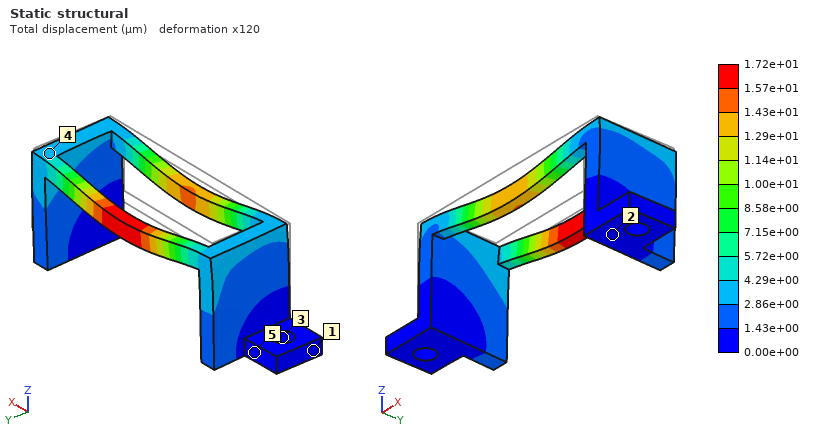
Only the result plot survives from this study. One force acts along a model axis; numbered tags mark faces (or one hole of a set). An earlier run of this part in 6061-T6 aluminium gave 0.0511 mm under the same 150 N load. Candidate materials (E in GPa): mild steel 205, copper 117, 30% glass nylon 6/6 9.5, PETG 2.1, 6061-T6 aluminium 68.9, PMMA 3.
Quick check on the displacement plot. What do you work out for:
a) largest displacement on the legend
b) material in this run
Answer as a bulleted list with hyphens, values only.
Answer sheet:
- 1.72e+01 µm
- mild steel
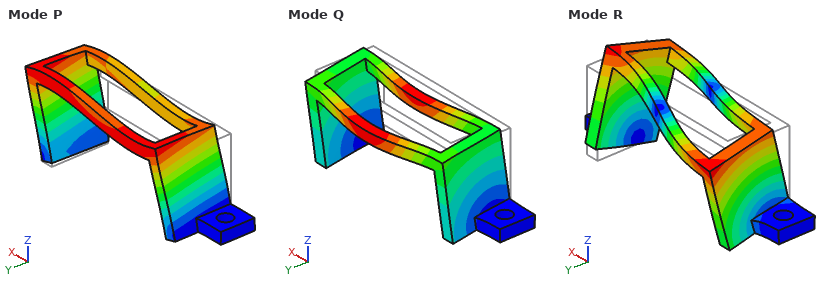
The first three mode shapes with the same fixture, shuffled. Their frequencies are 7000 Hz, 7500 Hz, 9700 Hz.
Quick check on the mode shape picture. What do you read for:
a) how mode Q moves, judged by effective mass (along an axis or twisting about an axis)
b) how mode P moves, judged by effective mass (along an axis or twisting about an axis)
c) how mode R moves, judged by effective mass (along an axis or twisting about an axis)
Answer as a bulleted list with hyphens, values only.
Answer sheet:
- along Y
- along X
- twisting about Z
